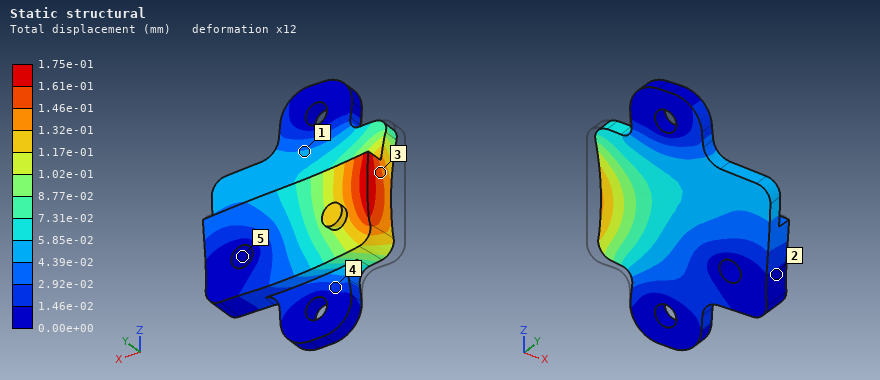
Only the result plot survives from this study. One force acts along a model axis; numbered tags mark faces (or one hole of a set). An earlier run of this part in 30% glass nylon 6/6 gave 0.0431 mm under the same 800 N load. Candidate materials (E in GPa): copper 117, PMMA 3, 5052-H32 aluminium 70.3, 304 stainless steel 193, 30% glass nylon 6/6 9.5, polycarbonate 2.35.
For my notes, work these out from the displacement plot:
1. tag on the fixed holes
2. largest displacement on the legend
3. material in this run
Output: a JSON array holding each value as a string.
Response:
["5", "1.75e-01 mm", "polycarbonate"]
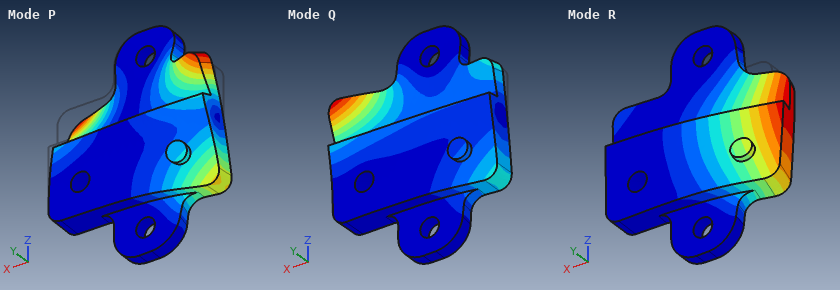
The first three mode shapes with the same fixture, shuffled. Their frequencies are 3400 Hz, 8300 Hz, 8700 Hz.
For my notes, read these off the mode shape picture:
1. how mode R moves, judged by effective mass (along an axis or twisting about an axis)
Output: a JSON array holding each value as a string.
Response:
["along Y"]
